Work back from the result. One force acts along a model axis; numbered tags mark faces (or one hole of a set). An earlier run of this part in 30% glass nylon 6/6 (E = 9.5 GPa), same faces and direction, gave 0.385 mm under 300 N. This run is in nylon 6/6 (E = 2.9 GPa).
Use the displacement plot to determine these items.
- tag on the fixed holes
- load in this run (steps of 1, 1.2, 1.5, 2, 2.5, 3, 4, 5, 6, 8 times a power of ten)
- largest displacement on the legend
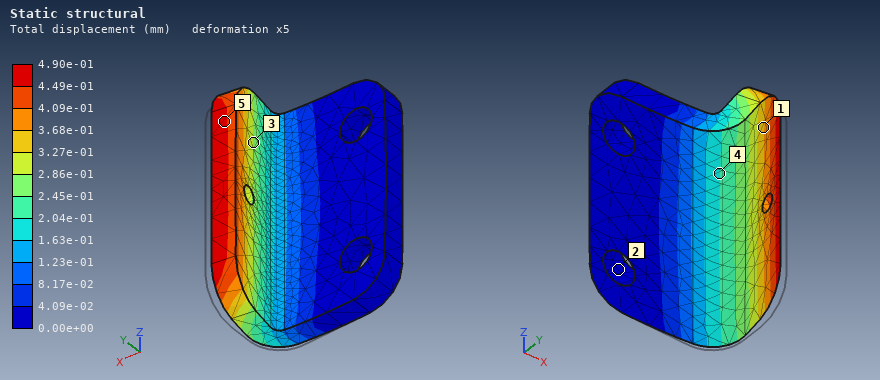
2
120 N
4.90e-01 mm
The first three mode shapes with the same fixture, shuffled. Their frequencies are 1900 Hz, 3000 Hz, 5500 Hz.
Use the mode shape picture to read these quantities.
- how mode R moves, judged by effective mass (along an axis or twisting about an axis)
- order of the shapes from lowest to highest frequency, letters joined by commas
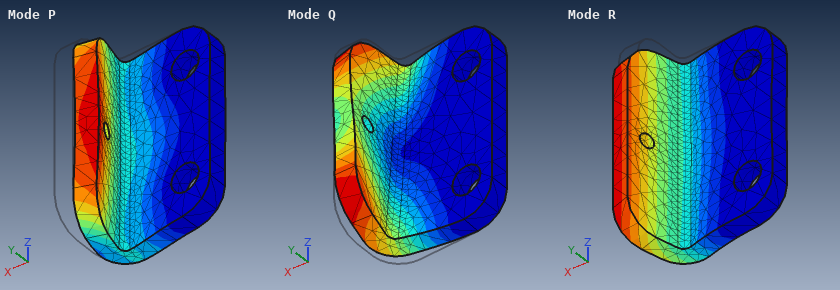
along Y
R, Q, P
